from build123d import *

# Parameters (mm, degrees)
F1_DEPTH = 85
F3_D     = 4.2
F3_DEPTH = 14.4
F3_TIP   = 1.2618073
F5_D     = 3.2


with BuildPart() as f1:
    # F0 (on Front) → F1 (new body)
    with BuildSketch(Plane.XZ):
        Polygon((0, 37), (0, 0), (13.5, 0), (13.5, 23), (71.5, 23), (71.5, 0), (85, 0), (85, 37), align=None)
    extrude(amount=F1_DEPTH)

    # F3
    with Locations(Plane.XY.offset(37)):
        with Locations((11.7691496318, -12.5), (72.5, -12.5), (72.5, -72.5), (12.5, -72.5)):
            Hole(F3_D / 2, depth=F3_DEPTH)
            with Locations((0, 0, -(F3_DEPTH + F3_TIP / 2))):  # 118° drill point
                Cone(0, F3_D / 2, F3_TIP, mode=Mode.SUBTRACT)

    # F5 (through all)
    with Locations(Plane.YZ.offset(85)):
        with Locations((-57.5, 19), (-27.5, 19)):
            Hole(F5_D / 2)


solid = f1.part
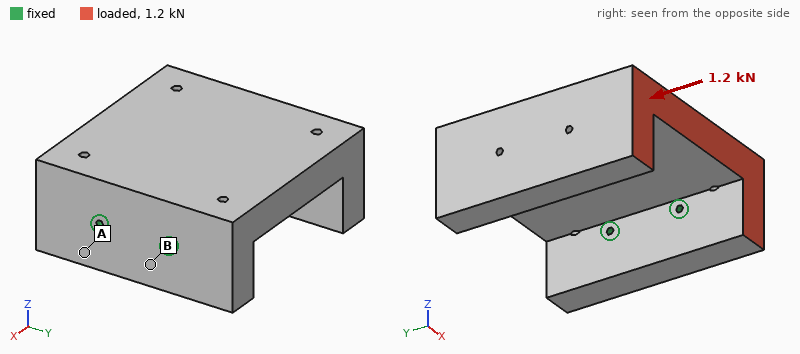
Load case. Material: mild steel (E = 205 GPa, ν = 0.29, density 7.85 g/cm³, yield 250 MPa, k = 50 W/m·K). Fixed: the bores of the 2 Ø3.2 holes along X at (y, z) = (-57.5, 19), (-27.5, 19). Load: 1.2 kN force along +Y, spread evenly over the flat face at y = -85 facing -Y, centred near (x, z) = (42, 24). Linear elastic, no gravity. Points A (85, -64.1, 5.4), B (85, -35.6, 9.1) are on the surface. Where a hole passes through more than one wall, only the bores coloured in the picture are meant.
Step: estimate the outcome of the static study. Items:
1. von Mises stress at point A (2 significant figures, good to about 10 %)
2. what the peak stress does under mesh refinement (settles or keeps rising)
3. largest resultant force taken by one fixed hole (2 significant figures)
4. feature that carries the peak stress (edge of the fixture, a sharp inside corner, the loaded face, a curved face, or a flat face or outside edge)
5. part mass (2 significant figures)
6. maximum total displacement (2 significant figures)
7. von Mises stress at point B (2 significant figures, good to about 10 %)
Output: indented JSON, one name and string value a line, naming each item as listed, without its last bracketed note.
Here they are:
{
  "von Mises stress at point A": "3.3 MPa",
  "what the peak stress does under mesh refinement": "keeps rising",
  "largest resultant force taken by one fixed hole": "1.3 kN",
  "feature that carries the peak stress": "edge of the fixture",
  "part mass": "1.2 kg",
  "maximum total displacement": "8.4 µm",
  "von Mises stress at point B": "1.6 MPa"
}
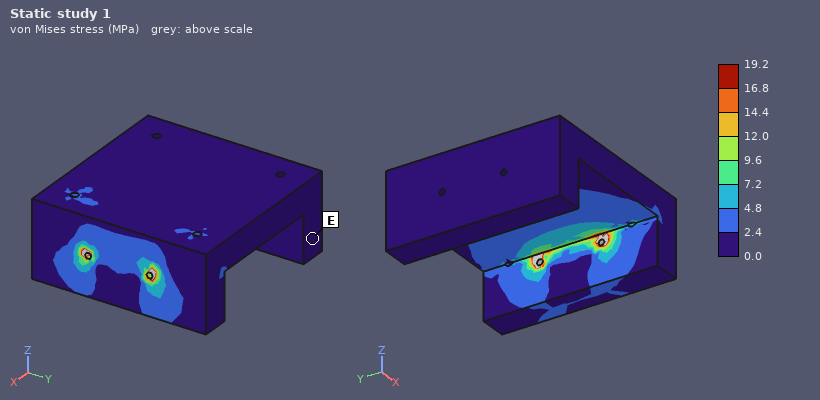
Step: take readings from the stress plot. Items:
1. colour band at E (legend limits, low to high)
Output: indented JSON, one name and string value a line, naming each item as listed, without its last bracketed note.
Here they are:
{
  "colour band at E": "0.0 to 2.4 MPa"
}
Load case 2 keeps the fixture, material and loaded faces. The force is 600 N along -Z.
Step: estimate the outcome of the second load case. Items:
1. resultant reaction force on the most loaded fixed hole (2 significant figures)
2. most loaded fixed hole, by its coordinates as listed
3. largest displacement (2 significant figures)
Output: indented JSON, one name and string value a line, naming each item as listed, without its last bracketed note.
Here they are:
{
  "resultant reaction force on the most loaded fixed hole": "1.1 kN",
  "most loaded fixed hole, by its coordinates as listed": "(-57.5, 19)",
  "largest displacement": "25 µm"
}
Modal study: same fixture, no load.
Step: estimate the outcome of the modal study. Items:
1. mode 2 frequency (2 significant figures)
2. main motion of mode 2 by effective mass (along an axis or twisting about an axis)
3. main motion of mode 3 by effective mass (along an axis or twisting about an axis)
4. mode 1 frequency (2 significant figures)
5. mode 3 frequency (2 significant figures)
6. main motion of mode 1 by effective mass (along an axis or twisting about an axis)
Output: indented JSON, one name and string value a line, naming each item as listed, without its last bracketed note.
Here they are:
{
  "mode 2 frequency": "2000 Hz",
  "main motion of mode 2 by effective mass": "along Y",
  "main motion of mode 3 by effective mass": "along Y",
  "mode 1 frequency": "960 Hz",
  "mode 3 frequency": "3000 Hz",
  "main motion of mode 1 by effective mass": "along Z"
}
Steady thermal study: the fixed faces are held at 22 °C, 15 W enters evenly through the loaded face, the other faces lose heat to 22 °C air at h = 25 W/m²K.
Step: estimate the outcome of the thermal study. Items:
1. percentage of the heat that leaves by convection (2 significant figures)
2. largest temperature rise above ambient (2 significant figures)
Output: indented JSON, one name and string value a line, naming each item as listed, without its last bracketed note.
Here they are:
{
  "percentage of the heat that leaves by convection": "28 %",
  "largest temperature rise above ambient": "14 K"
}
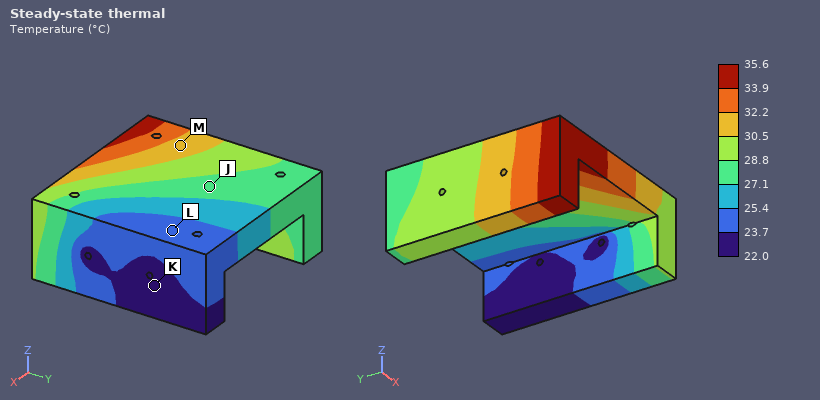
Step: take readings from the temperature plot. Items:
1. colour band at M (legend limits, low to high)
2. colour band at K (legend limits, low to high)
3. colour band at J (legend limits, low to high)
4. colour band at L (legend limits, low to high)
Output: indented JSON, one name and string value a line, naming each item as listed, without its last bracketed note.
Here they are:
{
  "colour band at M": "30.5 to 32.2 °C",
  "colour band at K": "22.0 to 23.7 °C",
  "colour band at J": "27.1 to 28.8 °C",
  "colour band at L": "23.7 to 25.4 °C"
}
